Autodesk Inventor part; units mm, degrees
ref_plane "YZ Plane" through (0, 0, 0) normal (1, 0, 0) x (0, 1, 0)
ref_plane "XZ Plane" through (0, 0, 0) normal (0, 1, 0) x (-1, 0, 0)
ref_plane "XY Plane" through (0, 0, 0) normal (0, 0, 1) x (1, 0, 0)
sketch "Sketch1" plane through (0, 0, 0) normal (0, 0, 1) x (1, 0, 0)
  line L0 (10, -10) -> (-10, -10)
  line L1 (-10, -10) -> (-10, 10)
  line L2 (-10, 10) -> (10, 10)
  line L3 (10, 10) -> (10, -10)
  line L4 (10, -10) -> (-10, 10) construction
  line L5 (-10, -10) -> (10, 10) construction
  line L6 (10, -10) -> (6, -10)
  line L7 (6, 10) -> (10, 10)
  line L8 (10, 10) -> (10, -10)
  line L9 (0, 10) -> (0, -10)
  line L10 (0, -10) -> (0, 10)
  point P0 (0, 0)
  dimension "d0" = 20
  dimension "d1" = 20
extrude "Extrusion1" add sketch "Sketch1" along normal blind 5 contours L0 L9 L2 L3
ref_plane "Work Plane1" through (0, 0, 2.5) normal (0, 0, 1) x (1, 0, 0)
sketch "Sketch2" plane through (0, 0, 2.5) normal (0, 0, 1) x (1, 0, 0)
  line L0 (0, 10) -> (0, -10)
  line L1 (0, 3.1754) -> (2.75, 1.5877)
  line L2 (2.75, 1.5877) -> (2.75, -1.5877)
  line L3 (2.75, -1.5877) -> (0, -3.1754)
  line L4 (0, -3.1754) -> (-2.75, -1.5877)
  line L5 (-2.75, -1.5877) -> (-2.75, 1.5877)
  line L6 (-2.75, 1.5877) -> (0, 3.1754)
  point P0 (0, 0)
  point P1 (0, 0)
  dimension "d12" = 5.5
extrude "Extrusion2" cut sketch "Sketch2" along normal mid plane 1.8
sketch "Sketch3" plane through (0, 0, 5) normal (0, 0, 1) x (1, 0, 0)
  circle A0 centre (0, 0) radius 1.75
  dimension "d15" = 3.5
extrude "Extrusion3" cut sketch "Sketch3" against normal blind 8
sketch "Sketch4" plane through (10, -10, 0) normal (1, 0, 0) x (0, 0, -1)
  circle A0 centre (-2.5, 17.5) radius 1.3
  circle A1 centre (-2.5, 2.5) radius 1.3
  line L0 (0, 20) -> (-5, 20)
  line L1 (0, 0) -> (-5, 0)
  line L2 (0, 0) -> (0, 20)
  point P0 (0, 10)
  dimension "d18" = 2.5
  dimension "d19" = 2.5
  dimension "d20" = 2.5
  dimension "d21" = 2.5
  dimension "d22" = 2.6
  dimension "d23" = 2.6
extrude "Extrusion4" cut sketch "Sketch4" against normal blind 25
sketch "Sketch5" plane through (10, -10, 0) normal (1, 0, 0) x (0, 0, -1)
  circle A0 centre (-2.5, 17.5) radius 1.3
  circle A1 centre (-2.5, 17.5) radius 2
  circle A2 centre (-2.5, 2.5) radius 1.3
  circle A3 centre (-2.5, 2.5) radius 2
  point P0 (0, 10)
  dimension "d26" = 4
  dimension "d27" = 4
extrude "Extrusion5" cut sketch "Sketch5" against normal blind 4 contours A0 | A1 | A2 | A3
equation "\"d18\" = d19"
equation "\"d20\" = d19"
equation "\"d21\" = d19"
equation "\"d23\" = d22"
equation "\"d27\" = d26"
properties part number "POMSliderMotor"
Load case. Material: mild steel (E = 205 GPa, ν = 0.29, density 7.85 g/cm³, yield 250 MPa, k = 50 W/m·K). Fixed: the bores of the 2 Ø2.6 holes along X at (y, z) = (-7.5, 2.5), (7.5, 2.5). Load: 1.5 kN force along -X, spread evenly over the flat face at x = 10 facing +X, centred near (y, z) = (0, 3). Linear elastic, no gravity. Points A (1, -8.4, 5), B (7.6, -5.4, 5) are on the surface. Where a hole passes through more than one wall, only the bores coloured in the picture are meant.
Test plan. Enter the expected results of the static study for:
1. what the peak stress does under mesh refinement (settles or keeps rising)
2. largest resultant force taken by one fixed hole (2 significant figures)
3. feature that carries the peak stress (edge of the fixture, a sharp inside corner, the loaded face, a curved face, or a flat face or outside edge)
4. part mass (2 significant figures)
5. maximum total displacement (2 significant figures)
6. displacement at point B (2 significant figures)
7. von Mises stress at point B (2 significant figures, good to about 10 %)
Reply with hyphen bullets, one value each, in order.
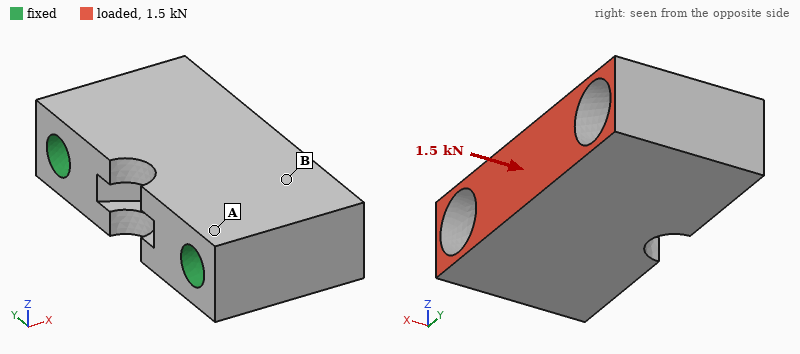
- keeps rising
- 800 N
- edge of the fixture
- 6.3 g
- 1.4 µm
- 0.78 µm
- 26 MPa
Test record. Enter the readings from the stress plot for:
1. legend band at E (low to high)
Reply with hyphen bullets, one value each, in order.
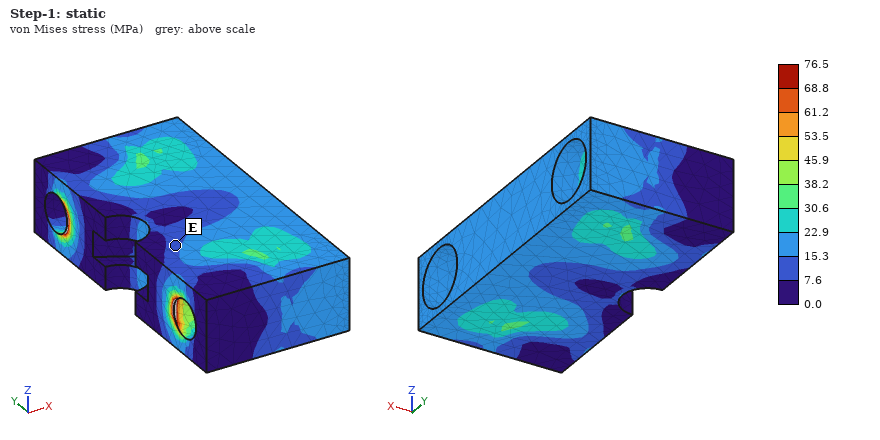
- 7.6 to 15.3 MPa
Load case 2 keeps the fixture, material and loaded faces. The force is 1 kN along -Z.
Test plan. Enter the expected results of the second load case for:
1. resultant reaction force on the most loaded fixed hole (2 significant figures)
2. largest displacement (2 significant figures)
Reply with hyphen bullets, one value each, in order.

- 500 N
- 8.0 µm
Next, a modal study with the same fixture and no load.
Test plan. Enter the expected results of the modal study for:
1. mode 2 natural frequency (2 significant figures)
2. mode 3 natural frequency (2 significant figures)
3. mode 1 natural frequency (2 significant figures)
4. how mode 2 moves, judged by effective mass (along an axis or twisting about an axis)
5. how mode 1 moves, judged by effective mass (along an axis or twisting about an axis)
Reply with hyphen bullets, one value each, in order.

- 88 kHz
- 93 kHz
- 51 kHz
- along X
- along Z
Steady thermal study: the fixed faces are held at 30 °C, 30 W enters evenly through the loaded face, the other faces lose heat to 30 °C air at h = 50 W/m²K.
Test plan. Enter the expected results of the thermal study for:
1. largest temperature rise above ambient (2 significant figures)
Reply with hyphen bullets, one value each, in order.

- 62 K
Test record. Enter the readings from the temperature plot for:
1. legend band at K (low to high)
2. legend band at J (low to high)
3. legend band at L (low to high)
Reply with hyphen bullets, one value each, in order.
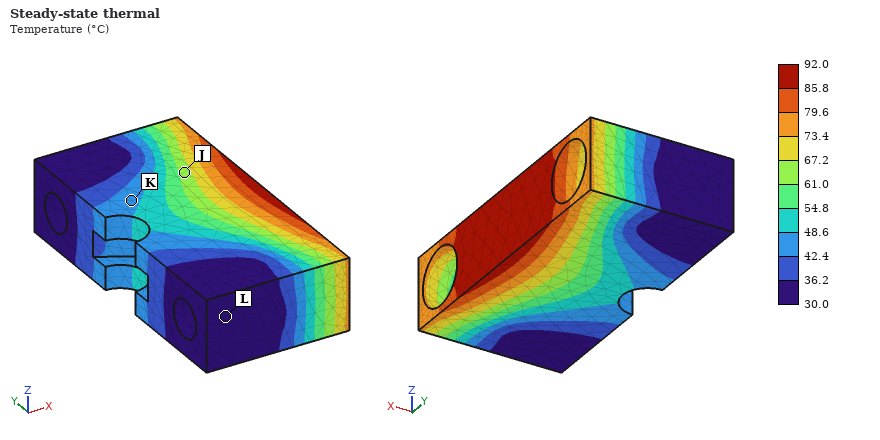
- 42.4 to 48.6 °C
- 61.0 to 67.2 °C
- 30.0 to 36.2 °C
